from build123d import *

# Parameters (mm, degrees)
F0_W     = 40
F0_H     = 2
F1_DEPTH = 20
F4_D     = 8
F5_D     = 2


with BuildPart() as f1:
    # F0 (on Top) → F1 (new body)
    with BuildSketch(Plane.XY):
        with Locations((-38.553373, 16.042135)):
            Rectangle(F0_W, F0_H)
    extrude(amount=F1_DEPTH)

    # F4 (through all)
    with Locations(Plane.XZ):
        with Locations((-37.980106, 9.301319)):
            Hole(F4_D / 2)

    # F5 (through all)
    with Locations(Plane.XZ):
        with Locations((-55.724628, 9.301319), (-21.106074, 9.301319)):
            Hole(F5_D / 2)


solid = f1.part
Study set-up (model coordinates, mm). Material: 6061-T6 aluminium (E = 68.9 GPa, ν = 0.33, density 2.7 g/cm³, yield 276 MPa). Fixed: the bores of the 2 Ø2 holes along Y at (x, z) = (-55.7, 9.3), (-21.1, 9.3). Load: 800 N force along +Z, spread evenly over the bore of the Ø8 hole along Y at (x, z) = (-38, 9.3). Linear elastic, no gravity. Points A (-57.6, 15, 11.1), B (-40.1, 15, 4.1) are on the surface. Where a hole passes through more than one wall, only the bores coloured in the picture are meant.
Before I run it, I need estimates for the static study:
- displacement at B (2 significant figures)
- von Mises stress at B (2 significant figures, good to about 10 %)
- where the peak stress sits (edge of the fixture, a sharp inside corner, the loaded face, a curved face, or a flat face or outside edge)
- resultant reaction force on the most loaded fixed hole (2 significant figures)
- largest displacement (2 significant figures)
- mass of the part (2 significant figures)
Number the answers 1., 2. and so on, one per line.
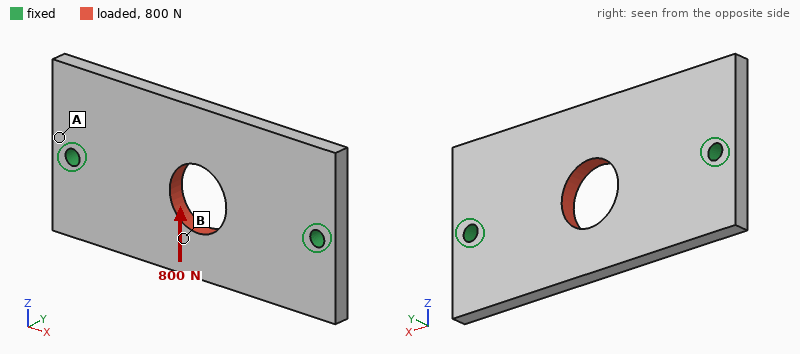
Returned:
1. 14 µm
2. 29 MPa
3. edge of the fixture
4. 410 N
5. 15 µm
6. 4.0 g
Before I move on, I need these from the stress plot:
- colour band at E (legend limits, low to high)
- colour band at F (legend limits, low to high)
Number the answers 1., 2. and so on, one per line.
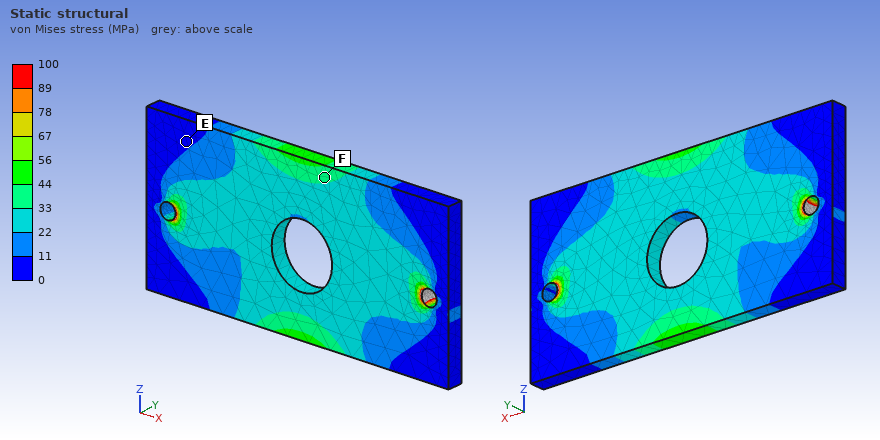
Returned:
1. 0 to 11 MPa
2. 33 to 44 MPa
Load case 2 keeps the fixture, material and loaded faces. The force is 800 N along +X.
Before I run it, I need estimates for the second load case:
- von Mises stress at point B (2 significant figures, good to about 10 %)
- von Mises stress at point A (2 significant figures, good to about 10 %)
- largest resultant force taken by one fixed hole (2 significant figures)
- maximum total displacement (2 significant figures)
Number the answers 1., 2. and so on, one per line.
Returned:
1. 9.7 MPa
2. 16 MPa
3. 400 N
4. 4.9 µm
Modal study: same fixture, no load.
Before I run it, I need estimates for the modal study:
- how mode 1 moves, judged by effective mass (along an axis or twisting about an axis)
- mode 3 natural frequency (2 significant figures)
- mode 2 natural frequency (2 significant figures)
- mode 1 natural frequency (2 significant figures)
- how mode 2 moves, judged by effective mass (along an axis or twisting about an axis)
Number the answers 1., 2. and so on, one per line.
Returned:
1. along Y
2. 14 kHz
3. 7700 Hz
4. 6800 Hz
5. along Y
